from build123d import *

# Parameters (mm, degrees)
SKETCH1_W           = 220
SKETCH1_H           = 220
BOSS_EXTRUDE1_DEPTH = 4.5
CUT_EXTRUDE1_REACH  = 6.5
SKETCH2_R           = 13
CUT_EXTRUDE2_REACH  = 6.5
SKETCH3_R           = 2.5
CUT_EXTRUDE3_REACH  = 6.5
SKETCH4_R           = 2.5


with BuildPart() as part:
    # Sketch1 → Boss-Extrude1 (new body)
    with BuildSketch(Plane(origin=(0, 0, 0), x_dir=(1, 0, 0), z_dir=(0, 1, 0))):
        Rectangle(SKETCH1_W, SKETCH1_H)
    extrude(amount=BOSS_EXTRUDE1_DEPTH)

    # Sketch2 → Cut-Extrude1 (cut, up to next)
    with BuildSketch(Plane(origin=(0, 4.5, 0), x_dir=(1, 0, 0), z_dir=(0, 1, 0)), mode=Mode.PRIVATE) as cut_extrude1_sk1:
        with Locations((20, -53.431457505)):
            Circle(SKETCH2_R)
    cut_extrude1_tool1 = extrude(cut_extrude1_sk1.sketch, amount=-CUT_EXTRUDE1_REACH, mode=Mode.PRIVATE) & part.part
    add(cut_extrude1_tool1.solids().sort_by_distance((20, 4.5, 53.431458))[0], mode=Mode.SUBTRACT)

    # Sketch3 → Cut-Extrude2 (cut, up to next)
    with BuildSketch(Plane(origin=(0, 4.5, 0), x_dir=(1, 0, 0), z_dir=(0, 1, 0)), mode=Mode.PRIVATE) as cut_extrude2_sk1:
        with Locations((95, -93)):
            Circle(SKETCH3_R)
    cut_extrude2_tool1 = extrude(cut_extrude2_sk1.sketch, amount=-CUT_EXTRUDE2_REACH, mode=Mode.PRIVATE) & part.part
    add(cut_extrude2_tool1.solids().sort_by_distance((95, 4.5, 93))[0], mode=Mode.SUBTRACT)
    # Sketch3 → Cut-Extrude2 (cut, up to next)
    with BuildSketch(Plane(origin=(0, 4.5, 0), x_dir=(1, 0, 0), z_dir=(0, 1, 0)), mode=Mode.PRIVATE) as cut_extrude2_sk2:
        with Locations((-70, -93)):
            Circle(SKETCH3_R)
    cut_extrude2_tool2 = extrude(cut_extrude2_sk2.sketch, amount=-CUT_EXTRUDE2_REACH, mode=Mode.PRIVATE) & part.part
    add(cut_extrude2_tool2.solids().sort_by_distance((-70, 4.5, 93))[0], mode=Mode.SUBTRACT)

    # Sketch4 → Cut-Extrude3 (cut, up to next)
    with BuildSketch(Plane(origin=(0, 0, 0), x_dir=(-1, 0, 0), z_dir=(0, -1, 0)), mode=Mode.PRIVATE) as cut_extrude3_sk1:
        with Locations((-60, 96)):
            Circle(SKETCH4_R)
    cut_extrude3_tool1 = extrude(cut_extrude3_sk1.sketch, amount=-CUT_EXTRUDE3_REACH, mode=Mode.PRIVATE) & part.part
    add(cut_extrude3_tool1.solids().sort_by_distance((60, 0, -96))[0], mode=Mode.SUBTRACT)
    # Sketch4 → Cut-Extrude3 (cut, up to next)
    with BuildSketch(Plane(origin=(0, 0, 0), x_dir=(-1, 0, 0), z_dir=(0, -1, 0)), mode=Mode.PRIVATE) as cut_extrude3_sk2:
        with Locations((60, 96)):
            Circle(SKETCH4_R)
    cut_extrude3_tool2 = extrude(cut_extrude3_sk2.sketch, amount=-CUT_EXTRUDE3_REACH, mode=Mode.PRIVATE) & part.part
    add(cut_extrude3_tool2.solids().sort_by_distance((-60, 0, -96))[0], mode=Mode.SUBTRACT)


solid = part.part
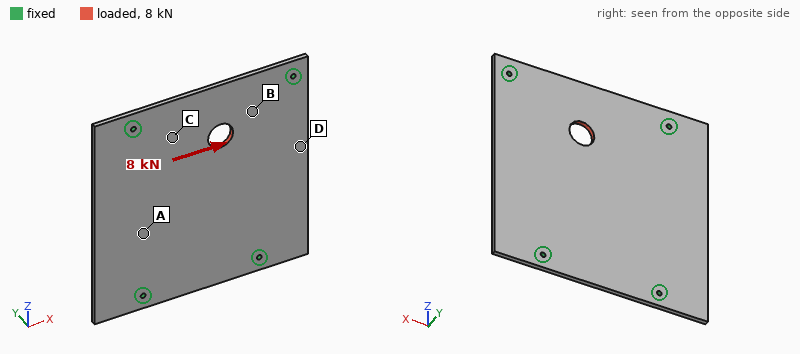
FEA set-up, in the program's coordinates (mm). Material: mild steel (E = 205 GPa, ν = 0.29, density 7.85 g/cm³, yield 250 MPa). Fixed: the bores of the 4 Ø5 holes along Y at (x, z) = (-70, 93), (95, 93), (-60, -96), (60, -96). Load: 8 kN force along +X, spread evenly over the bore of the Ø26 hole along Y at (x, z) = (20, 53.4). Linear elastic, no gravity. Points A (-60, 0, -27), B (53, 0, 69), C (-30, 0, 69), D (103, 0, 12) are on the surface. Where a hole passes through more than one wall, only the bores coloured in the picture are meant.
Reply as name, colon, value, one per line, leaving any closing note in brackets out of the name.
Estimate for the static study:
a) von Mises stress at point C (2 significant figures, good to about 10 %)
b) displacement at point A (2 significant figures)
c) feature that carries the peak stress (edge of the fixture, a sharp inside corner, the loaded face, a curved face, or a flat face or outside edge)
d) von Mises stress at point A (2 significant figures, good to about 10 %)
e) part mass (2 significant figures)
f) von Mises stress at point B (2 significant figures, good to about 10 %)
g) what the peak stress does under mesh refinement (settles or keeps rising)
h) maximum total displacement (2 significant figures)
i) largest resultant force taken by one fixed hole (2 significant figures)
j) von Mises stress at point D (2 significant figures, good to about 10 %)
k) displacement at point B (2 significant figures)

von Mises stress at point C: 14 MPa
displacement at point A: 3.7 µm
feature that carries the peak stress: edge of the fixture
von Mises stress at point A: 3.9 MPa
part mass: 1.7 kg
von Mises stress at point B: 16 MPa
what the peak stress does under mesh refinement: keeps rising
maximum total displacement: 9.0 µm
largest resultant force taken by one fixed hole: 3.1 kN
von Mises stress at point D: 6.2 MPa
displacement at point B: 5.8 µm
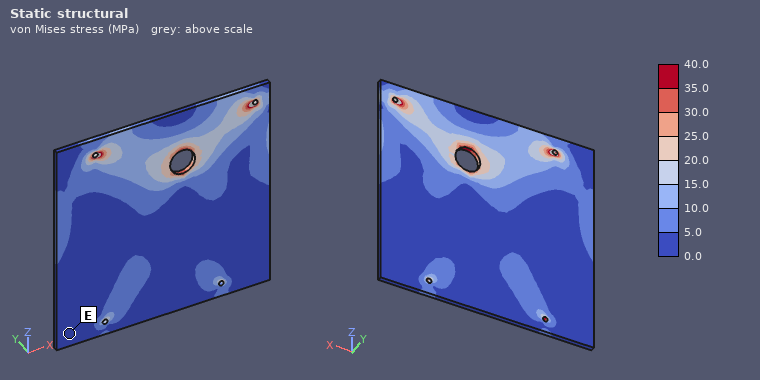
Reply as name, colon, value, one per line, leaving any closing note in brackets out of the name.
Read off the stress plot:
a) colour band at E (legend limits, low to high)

colour band at E: 0.0 to 5.0 MPa
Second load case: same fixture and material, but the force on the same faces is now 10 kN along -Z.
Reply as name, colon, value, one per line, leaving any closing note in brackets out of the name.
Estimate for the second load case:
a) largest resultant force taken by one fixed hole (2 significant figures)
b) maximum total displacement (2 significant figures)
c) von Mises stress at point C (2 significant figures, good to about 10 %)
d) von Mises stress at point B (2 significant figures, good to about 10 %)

largest resultant force taken by one fixed hole: 2.9 kN
maximum total displacement: 14 µm
von Mises stress at point C: 13 MPa
von Mises stress at point B: 14 MPa
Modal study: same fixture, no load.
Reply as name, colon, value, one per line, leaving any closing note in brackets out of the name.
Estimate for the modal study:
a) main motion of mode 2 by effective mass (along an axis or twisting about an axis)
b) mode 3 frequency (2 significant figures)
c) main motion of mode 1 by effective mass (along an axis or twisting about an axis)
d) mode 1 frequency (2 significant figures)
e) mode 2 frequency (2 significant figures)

main motion of mode 2 by effective mass: twisting about Z
mode 3 frequency: 760 Hz
main motion of mode 1 by effective mass: along Y
mode 1 frequency: 490 Hz
mode 2 frequency: 620 Hz
